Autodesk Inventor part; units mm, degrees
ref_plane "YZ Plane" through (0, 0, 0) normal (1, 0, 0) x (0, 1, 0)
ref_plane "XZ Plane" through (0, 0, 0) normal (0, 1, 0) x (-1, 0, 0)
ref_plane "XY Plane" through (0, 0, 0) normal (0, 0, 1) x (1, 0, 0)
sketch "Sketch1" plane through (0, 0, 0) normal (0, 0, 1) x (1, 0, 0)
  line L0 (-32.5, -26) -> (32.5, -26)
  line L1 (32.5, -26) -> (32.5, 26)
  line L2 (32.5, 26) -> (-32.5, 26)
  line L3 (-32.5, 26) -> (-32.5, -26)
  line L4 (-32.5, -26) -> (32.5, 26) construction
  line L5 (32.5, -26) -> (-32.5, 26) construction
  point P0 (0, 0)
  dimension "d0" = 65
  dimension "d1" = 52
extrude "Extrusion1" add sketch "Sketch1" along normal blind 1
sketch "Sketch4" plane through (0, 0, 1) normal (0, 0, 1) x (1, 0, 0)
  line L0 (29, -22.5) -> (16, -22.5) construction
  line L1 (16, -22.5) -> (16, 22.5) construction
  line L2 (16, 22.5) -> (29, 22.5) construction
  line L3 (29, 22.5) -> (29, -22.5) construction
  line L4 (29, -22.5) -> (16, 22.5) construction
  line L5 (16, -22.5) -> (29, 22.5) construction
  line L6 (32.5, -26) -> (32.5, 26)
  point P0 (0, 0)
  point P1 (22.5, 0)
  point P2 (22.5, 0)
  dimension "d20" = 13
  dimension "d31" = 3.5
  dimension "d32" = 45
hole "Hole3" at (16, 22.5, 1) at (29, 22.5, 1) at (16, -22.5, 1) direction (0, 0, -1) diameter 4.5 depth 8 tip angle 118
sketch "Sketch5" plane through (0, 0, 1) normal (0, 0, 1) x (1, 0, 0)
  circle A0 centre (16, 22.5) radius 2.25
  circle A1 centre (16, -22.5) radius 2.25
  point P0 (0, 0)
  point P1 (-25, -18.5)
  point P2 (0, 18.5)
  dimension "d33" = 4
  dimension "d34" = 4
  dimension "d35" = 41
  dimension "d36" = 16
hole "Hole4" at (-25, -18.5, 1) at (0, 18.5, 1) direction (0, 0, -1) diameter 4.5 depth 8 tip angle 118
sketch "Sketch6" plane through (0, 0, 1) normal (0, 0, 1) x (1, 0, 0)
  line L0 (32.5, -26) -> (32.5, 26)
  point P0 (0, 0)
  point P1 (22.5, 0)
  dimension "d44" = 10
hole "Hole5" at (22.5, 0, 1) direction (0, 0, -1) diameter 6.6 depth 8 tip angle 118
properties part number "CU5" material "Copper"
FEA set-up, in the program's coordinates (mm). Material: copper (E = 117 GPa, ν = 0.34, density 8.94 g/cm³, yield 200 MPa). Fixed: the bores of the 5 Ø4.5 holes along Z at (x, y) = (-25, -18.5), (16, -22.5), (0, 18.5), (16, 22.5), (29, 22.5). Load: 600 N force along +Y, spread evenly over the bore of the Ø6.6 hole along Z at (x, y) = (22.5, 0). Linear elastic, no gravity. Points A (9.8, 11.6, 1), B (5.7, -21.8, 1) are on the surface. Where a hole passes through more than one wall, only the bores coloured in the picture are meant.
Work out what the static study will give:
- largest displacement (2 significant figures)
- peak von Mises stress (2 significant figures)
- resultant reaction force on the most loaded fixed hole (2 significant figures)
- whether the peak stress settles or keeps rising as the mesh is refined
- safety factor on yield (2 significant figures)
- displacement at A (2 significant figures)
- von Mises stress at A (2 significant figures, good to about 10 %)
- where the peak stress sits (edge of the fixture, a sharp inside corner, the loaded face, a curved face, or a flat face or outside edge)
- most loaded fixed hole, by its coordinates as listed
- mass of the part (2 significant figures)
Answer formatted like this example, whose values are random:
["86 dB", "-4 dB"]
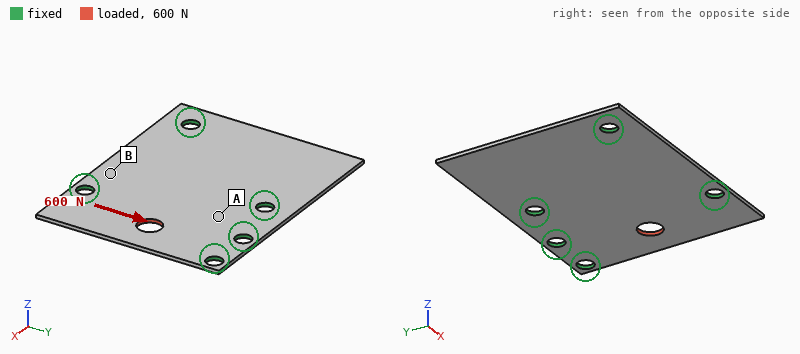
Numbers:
["4.2 µm", "51 MPa", "220 N", "settles", "3.9", "0.75 µm", "7.4 MPa", "the loaded face", "(16, -22.5)", "29 g"]
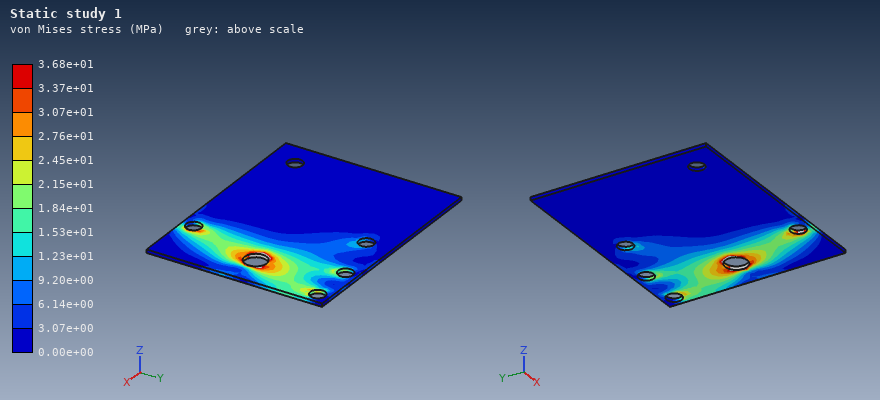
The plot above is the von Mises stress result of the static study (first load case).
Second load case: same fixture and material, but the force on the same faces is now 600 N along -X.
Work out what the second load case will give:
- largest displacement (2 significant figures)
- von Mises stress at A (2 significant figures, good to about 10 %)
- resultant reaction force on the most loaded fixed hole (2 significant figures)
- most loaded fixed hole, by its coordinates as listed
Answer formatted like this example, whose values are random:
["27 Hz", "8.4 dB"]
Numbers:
["6.8 µm", "17 MPa", "190 N", "(0, 18.5)"]
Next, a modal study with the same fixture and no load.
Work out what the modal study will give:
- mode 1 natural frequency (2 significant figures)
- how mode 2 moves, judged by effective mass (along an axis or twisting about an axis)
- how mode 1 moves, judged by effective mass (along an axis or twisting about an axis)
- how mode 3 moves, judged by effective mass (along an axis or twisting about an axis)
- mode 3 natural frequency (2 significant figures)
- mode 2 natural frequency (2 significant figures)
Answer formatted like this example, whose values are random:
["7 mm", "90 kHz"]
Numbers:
["910 Hz", "along Z", "along Z", "along Z", "2100 Hz", "1900 Hz"]
